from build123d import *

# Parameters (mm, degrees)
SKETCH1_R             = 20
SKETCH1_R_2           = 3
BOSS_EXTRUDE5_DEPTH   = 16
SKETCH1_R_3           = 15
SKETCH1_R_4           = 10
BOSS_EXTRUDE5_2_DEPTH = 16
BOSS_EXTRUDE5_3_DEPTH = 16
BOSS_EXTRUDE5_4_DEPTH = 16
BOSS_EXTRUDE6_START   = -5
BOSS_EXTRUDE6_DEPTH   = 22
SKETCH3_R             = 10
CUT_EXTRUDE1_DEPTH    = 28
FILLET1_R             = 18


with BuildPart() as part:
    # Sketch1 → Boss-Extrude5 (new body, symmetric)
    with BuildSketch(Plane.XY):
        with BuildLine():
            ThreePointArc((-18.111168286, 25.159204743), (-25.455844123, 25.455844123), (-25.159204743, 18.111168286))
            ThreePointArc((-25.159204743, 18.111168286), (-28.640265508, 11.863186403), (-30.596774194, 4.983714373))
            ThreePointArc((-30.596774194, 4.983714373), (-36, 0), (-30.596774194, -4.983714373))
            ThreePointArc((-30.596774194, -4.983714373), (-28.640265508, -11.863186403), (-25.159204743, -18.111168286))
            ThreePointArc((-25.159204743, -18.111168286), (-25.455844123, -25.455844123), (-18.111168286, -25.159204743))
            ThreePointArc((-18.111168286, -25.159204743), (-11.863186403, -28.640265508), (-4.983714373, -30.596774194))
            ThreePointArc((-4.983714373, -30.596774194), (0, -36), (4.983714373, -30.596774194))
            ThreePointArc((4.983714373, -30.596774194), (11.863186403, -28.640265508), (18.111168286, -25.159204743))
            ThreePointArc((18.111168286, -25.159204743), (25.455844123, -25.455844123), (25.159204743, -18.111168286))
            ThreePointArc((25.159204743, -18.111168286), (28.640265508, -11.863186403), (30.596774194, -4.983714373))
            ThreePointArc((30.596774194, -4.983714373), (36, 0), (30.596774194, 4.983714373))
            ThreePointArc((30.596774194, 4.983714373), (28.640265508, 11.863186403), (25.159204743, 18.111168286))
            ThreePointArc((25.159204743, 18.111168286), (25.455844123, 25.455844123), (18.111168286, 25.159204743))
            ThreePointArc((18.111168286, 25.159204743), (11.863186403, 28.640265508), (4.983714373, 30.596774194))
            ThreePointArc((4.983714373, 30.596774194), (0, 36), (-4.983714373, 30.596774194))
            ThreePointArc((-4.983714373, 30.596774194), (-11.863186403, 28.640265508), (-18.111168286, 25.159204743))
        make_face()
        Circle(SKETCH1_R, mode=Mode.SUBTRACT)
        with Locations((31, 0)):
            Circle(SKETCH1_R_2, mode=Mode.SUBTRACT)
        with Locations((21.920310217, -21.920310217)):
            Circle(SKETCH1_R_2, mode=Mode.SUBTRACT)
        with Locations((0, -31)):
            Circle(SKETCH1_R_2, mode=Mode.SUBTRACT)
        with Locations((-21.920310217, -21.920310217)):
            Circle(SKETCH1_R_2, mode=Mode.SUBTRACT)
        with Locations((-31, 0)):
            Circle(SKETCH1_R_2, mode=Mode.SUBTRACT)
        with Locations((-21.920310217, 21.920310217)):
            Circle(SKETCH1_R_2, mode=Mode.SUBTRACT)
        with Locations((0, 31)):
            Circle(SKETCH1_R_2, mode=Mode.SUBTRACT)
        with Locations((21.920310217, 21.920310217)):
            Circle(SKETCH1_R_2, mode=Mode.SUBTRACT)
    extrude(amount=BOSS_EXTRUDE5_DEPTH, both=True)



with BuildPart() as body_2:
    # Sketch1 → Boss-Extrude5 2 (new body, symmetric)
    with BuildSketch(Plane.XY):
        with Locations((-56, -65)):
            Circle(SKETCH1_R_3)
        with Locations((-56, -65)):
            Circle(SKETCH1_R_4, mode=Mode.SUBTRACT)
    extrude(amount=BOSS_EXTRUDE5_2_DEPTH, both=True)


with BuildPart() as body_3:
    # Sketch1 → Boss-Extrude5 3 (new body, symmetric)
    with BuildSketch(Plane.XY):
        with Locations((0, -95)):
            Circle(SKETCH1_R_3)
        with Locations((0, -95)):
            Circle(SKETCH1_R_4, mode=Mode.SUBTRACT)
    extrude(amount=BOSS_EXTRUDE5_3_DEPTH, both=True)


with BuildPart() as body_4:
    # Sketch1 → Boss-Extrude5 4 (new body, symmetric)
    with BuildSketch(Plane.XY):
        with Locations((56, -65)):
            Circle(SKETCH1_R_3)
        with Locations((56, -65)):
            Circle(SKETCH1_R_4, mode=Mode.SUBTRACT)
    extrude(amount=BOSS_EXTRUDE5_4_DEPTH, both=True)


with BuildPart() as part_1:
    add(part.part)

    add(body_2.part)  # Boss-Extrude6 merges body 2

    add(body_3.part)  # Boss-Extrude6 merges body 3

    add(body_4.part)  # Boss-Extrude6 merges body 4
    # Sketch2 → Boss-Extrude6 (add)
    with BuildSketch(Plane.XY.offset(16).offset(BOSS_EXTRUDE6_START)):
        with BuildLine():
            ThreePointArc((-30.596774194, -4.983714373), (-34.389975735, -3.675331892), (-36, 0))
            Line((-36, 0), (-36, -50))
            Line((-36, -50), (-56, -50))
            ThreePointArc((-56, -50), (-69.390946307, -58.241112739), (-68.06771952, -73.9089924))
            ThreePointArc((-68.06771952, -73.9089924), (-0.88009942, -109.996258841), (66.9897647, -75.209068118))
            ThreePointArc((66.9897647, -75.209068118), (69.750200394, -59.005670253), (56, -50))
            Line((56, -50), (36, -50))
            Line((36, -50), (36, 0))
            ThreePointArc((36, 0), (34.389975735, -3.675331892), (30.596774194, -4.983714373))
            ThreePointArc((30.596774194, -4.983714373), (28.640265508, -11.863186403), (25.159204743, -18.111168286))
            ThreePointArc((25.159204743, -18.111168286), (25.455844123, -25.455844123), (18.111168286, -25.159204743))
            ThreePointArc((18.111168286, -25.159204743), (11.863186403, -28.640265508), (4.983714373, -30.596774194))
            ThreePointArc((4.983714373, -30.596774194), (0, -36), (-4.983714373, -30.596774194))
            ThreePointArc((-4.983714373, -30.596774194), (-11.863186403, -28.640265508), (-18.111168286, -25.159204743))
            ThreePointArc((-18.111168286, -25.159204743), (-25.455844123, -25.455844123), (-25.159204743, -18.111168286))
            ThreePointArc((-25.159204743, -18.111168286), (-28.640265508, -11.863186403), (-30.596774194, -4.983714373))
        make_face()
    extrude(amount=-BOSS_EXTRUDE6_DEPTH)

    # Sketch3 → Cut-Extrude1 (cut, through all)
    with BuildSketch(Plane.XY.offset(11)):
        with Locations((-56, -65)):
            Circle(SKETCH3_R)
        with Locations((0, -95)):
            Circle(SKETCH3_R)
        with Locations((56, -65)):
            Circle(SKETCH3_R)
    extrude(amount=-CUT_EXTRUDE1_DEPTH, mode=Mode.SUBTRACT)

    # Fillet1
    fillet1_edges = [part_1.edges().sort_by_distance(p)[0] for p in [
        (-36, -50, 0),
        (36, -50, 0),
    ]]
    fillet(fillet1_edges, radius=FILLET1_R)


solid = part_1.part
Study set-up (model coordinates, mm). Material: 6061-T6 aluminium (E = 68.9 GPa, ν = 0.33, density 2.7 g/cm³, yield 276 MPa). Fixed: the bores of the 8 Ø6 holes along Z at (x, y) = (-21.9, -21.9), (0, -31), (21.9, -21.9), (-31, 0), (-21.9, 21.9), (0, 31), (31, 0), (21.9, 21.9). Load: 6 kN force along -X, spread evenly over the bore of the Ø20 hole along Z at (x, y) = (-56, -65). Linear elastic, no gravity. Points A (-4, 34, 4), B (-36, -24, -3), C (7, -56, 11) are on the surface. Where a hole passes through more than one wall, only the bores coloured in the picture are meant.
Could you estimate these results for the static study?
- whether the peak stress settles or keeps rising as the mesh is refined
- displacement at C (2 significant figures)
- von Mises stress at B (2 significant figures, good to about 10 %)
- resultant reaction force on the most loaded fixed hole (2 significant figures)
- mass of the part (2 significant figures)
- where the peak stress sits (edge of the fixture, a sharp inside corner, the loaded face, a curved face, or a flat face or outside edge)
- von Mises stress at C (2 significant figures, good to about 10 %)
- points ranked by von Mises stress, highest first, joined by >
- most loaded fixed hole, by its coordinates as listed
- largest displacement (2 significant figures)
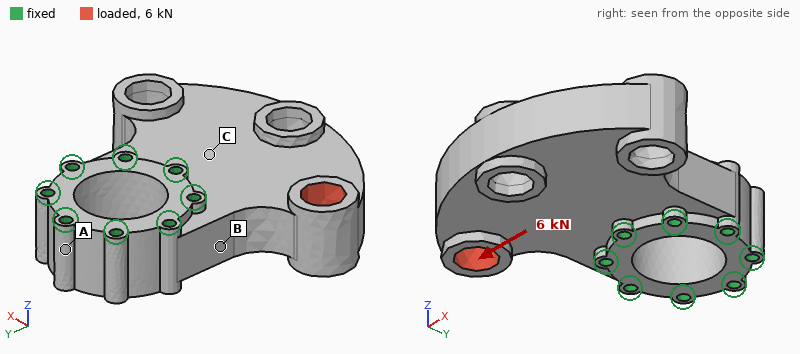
keeps rising
6.7 µm
11 MPa
4.4 kN
660 g
edge of the fixture
6.3 MPa
B > C > A
(0, -31)
21 µm
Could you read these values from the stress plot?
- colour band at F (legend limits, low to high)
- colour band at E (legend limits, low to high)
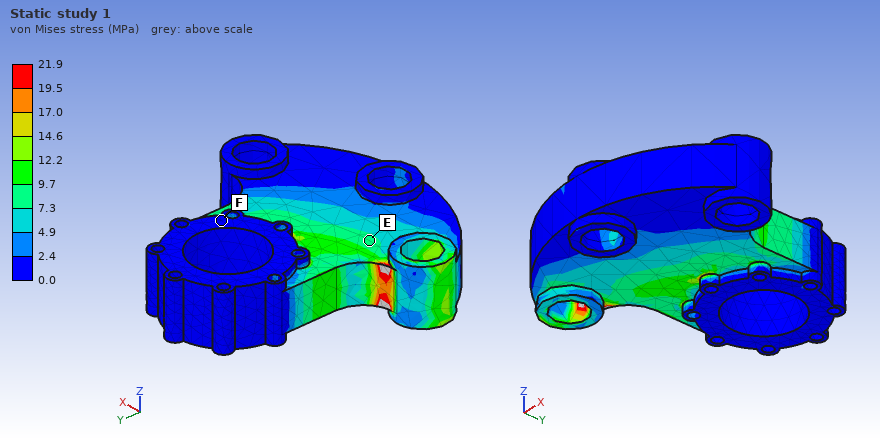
0.0 to 2.4 MPa
7.3 to 9.7 MPa
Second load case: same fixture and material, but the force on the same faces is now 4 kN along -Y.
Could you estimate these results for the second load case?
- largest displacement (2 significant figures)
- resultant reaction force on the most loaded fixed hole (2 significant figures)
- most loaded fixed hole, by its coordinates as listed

29 µm
4.7 kN
(-21.9, -21.9)
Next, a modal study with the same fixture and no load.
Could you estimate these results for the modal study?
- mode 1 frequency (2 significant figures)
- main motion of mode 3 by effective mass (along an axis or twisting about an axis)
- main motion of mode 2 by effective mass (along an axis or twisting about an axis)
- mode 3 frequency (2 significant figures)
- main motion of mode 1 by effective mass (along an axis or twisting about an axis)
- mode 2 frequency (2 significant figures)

2400 Hz
along X
twisting about Y
4300 Hz
along Z
3200 Hz
